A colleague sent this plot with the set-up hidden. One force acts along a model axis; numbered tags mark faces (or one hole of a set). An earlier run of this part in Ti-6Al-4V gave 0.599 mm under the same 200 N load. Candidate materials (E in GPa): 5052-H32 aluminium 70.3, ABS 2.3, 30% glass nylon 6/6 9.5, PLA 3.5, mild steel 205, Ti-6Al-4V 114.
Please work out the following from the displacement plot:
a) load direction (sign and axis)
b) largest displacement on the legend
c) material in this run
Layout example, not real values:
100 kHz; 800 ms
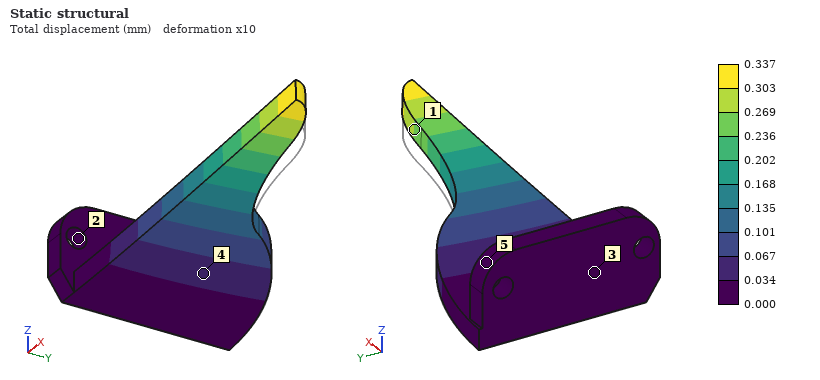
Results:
+Z; 0.337 mm; mild steel
